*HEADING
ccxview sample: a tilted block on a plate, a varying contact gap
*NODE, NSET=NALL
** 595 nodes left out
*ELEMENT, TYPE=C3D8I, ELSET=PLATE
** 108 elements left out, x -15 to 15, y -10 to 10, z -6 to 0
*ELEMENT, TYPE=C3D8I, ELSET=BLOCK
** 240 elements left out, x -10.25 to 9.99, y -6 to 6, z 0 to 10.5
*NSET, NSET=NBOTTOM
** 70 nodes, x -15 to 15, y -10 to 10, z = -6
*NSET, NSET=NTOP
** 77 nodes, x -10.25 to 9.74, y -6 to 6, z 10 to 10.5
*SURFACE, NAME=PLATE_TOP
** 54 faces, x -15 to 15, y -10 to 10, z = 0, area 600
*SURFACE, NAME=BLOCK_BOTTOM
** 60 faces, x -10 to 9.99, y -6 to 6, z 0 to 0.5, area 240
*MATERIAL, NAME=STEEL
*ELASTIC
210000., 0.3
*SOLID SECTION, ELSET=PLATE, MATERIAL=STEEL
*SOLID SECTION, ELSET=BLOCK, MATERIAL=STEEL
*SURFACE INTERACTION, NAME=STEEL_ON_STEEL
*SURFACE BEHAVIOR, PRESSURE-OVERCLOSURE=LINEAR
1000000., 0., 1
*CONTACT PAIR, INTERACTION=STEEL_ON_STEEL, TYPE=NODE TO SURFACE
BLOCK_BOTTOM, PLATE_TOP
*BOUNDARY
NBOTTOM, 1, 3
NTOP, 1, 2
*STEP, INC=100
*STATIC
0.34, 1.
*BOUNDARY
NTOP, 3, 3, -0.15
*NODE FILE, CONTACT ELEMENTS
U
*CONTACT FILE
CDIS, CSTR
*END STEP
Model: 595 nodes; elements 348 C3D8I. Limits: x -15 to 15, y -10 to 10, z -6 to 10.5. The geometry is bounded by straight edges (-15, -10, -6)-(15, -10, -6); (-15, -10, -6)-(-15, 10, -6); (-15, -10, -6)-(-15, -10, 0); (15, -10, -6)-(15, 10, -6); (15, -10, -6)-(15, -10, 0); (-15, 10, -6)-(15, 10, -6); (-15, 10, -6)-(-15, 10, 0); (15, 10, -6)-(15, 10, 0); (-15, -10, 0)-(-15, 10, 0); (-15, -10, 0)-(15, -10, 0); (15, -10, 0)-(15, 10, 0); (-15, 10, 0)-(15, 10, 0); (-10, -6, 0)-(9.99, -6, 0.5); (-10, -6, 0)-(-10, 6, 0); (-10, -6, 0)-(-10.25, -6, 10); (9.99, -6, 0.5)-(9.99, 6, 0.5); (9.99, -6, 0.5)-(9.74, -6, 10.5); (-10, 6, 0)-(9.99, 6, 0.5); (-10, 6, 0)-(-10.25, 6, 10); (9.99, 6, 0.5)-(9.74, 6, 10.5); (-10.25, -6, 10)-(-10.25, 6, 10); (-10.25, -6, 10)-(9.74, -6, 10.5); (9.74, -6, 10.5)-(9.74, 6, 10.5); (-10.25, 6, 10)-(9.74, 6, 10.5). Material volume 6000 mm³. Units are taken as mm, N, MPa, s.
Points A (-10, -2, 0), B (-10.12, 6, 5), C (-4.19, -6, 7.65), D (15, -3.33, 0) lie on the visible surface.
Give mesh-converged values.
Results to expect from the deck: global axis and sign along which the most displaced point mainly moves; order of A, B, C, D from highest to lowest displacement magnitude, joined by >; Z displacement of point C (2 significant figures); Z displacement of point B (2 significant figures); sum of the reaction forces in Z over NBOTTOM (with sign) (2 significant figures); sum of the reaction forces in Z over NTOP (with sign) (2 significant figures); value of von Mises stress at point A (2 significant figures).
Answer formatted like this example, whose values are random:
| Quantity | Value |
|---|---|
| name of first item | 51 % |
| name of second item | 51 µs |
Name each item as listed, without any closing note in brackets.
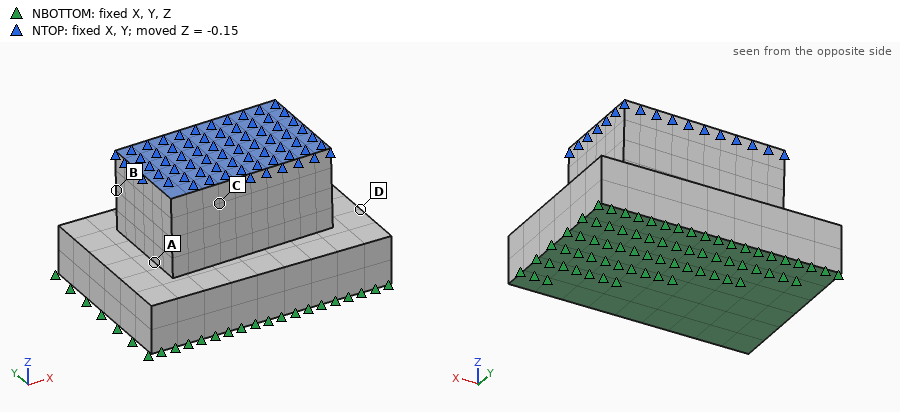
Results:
| Quantity | Value |
|---|---|
| global axis and sign along which the most displaced point mainly moves | -Z |
| order of A, B, C, D from highest to lowest displacement magnitude, joined by > | C > B > A > D |
| Z displacement of point C | -0.14 mm |
| Z displacement of point B | -0.10 mm |
| sum of the reaction forces in Z over NBOTTOM (with sign) | 91000 N |
| sum of the reaction forces in Z over NTOP (with sign) | -91000 N |
| value of von Mises stress at point A | 4300 MPa |
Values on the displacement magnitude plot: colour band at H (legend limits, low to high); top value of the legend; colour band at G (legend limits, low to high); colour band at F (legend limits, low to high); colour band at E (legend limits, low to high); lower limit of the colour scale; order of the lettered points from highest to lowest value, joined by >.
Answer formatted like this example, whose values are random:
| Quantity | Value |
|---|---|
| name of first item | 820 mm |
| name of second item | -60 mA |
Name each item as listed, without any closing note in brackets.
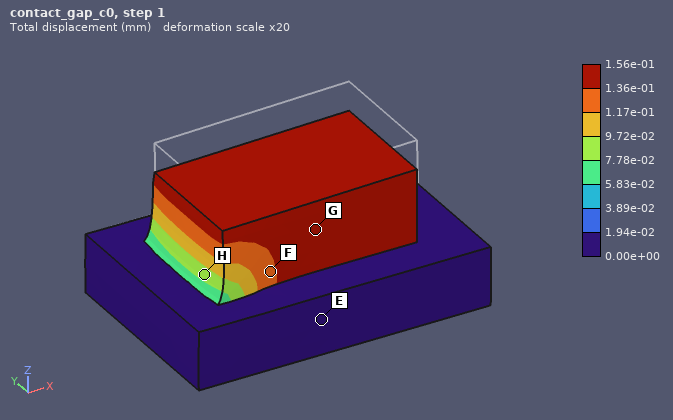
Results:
| Quantity | Value |
|---|---|
| colour band at H | 7.78e-02 to 9.72e-02 mm |
| top value of the legend | 1.56e-01 mm |
| colour band at G | 1.36e-01 to 1.56e-01 mm |
| colour band at F | 1.17e-01 to 1.36e-01 mm |
| colour band at E | 0.00e+00 to 1.94e-02 mm |
| lower limit of the colour scale | 0.00e+00 mm |
| order of the lettered points from highest to lowest value, joined by > | G > F > H > E |
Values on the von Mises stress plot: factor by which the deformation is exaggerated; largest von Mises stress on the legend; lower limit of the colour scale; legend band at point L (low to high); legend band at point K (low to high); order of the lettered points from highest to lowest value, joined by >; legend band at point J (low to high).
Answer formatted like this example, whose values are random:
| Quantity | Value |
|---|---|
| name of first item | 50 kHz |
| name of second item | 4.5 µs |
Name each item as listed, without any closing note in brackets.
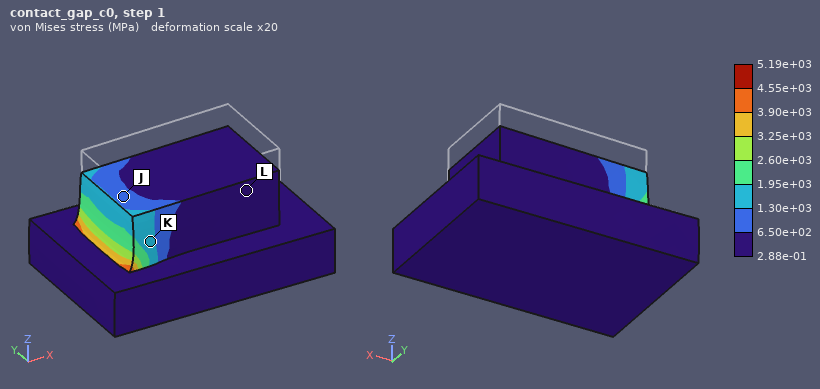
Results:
| Quantity | Value |
|---|---|
| factor by which the deformation is exaggerated | 20 |
| largest von Mises stress on the legend | 5.19e+03 MPa |
| lower limit of the colour scale | 2.88e-01 MPa |
| legend band at point L | 2.88e-01 to 6.50e+02 MPa |
| legend band at point K | 1.30e+03 to 1.95e+03 MPa |
| order of the lettered points from highest to lowest value, joined by > | K > J > L |
| legend band at point J | 6.50e+02 to 1.30e+03 MPa |
